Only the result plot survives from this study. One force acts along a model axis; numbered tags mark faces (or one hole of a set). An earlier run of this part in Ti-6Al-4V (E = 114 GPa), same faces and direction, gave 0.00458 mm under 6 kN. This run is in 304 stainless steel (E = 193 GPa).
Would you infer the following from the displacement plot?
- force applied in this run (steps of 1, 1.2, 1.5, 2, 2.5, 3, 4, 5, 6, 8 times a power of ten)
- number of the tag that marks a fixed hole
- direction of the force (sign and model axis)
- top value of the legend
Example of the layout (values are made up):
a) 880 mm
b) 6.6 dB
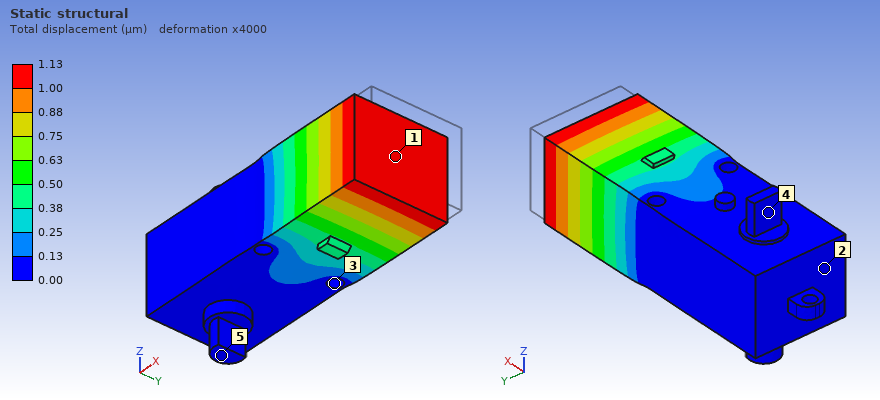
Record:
a) 2.5 kN
b) 3
c) -X
d) 1.13 µm
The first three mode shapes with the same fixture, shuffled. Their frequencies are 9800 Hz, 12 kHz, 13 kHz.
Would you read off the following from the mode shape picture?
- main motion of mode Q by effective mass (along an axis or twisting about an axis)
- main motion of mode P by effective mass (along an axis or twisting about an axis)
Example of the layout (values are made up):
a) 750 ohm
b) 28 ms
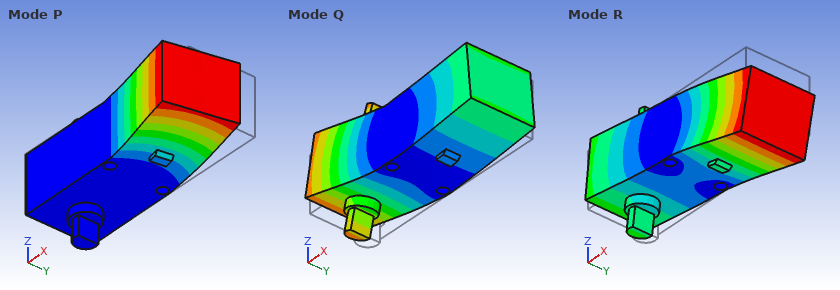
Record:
a) along Z
b) along Y
